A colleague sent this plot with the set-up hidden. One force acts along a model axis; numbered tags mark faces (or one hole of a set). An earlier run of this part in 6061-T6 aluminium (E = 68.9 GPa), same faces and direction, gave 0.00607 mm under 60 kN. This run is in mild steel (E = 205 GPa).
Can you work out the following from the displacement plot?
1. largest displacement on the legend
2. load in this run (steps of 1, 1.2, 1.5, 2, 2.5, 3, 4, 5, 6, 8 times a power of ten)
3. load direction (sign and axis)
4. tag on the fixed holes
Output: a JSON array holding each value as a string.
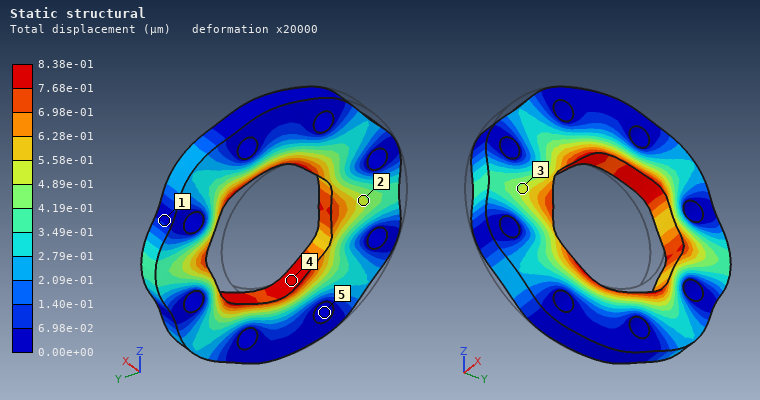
["8.38e-01 µm", "25 kN", "+Y", "5"]
